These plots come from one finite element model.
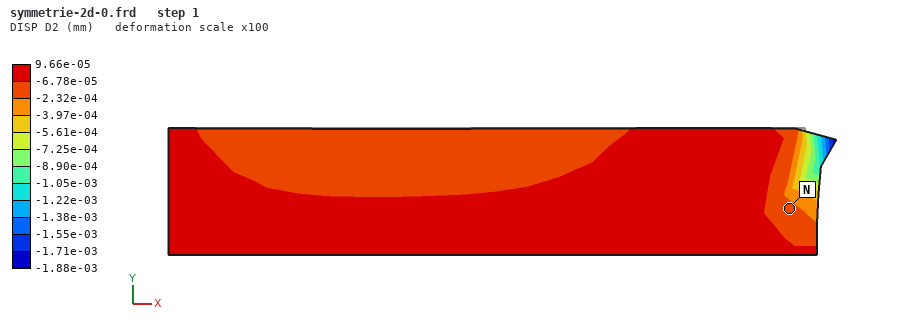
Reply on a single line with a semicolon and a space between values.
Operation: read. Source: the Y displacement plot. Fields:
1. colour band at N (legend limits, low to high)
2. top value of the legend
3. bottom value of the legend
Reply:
-2.32e-04 to -6.78e-05 mm; 9.66e-05 mm; -1.88e-03 mm
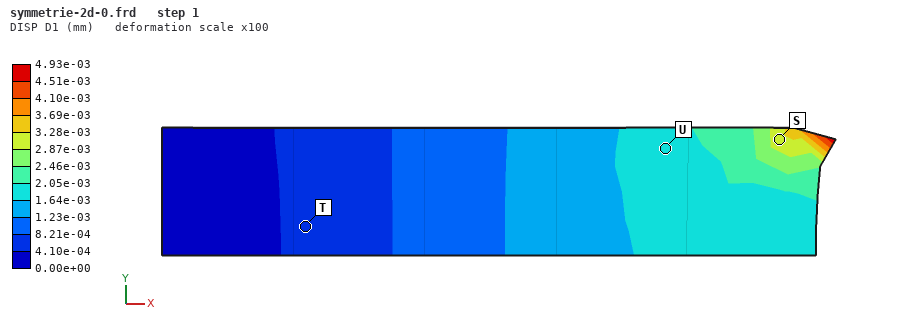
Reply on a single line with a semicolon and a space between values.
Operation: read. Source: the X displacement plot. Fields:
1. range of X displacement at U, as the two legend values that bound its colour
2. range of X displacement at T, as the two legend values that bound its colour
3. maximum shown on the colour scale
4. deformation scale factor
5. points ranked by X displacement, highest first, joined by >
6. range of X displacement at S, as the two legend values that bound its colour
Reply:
1.64e-03 to 2.05e-03 mm; 4.10e-04 to 8.21e-04 mm; 4.93e-03 mm; 100; S > U > T; 2.87e-03 to 3.28e-03 mm
